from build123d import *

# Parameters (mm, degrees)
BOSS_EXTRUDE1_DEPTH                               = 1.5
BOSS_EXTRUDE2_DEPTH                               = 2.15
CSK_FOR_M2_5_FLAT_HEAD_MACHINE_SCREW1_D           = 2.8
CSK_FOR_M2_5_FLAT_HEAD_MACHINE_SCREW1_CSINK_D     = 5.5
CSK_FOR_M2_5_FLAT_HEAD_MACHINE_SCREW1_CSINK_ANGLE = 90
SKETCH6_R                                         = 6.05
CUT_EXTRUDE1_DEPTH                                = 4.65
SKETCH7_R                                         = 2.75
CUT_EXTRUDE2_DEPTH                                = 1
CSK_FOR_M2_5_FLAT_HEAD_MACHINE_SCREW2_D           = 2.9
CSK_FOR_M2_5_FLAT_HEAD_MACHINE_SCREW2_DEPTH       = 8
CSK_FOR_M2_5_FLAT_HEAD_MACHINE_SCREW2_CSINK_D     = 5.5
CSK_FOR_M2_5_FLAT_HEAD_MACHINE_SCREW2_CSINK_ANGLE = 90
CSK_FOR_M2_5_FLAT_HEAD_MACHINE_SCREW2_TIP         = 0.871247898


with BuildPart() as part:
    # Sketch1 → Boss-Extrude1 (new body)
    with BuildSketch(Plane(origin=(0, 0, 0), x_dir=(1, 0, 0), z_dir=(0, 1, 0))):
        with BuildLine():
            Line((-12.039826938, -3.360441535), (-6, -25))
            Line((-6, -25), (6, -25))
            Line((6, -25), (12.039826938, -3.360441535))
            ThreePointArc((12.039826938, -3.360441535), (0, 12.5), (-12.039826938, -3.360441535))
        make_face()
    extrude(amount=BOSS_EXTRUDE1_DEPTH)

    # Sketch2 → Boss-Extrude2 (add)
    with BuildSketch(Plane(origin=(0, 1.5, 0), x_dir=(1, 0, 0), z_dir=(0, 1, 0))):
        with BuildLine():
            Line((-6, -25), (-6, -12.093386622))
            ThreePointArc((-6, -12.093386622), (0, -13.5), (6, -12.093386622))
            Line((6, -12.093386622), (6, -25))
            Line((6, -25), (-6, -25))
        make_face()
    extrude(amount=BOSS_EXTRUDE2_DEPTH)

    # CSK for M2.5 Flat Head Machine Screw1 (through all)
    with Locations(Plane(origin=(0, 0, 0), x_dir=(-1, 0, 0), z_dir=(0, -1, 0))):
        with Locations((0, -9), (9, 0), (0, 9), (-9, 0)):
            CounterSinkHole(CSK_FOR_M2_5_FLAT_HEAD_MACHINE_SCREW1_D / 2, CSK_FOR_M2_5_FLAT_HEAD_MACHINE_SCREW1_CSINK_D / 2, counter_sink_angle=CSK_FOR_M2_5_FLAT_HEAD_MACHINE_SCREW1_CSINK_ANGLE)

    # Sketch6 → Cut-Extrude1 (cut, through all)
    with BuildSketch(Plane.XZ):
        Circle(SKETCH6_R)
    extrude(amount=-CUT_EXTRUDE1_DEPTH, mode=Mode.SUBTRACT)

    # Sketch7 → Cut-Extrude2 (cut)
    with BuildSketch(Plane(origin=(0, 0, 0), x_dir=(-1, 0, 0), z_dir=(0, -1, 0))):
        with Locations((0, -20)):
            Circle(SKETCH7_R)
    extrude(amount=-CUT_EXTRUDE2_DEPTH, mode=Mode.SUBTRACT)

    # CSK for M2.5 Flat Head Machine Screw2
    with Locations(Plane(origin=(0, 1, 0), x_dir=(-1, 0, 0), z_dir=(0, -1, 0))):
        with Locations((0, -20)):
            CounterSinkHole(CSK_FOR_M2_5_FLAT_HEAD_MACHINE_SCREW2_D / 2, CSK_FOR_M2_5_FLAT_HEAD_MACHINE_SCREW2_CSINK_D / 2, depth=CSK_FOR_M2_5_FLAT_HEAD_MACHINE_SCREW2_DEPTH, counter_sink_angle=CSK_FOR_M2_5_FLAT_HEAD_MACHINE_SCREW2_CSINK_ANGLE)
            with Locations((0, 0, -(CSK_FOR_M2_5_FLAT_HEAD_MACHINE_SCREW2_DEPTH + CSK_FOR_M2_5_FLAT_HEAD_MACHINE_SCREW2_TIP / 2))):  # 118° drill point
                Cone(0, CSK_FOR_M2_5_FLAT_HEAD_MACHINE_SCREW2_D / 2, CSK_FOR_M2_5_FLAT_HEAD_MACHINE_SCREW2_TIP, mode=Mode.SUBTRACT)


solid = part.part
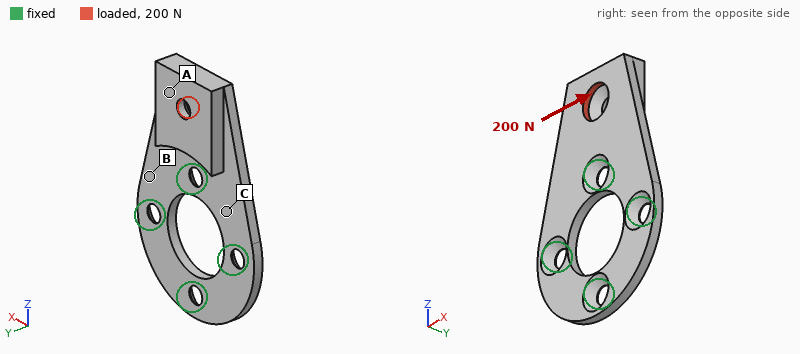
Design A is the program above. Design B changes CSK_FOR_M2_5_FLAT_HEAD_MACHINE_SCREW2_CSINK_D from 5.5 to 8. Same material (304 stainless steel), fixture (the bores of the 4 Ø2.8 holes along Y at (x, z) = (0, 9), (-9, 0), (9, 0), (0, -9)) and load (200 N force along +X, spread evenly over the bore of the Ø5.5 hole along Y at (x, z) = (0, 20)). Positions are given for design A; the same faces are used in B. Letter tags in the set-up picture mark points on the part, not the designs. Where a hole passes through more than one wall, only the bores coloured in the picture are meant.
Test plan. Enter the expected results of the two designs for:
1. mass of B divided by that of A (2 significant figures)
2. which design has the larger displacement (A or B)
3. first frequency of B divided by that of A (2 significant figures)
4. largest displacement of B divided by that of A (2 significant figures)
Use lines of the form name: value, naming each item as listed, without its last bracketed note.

mass of B divided by that of A: 0.94
which design has the larger displacement: B
first frequency of B divided by that of A: 1.1
largest displacement of B divided by that of A: 1.2
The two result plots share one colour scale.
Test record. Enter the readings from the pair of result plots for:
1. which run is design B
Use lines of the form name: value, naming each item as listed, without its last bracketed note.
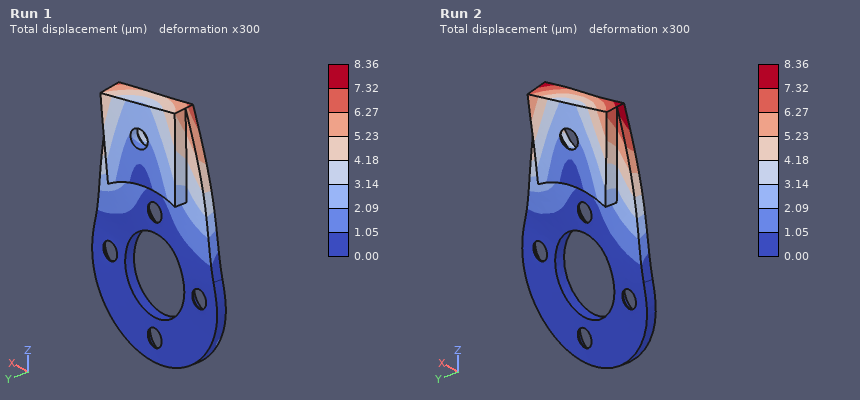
which run is design B: Run 2
